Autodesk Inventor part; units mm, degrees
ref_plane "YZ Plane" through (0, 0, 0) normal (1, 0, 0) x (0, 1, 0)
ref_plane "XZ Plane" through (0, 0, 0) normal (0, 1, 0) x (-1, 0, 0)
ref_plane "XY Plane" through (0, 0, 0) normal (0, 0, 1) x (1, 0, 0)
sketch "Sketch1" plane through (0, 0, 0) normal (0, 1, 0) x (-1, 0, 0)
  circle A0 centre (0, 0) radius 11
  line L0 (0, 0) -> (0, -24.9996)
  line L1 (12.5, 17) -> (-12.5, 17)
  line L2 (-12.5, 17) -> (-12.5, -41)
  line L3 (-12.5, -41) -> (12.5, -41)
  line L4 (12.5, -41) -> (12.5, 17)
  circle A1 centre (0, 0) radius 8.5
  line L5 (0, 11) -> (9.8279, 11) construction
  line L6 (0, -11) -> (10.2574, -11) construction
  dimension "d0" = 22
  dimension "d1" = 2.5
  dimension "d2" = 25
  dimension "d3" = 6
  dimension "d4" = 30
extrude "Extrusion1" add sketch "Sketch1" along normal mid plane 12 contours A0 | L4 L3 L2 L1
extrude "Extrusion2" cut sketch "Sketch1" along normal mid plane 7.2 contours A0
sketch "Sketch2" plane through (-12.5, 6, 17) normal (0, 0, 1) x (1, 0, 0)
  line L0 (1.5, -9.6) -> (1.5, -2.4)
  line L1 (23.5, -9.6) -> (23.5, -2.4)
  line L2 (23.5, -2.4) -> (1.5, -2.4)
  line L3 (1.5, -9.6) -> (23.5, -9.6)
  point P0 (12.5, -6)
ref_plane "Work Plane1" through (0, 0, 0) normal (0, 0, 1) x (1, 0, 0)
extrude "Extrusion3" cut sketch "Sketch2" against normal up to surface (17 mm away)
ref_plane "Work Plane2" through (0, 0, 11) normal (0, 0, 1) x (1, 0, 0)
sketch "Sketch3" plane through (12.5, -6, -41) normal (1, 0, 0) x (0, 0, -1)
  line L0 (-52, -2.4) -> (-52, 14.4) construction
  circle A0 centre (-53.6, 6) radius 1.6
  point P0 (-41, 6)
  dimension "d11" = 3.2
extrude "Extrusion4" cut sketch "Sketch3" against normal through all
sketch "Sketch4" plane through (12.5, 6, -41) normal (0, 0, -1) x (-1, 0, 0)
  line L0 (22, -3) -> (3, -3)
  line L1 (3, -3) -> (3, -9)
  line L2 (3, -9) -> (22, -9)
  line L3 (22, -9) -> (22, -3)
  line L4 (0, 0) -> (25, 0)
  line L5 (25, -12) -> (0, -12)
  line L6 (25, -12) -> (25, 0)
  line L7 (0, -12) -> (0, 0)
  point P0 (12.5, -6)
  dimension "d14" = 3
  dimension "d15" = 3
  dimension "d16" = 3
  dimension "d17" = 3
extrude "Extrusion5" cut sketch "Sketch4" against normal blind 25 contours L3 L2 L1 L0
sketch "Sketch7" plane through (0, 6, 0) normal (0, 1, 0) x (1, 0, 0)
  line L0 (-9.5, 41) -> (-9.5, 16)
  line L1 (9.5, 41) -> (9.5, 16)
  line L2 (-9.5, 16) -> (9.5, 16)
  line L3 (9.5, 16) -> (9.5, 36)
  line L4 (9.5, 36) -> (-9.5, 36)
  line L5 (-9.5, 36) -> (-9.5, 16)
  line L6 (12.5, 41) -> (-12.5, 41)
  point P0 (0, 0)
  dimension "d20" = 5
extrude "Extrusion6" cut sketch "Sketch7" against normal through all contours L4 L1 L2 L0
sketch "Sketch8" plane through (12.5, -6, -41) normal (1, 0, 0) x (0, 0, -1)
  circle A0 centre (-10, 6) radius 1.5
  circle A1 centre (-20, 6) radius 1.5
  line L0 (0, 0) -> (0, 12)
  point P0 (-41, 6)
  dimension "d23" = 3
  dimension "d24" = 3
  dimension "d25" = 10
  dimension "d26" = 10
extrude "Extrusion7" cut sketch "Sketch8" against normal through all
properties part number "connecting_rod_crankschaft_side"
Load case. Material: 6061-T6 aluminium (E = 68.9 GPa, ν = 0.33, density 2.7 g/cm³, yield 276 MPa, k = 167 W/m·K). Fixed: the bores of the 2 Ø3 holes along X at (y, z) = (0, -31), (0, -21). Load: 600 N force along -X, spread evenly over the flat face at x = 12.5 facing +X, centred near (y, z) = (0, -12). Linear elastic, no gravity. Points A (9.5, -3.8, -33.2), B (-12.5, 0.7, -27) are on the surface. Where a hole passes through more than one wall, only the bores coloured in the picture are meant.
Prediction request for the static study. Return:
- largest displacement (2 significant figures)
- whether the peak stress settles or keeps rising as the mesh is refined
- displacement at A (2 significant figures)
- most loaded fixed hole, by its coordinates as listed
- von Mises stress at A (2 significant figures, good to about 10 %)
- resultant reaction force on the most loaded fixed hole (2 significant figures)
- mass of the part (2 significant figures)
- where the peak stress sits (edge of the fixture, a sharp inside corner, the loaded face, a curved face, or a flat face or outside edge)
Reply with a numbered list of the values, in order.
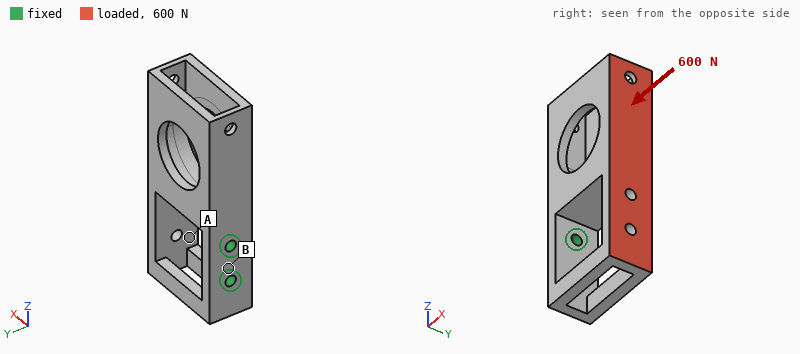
1. 0.29 mm
2. keeps rising
3. 0.13 mm
4. (0, -21)
5. 63 MPa
6. 710 N
7. 19 g
8. edge of the fixture
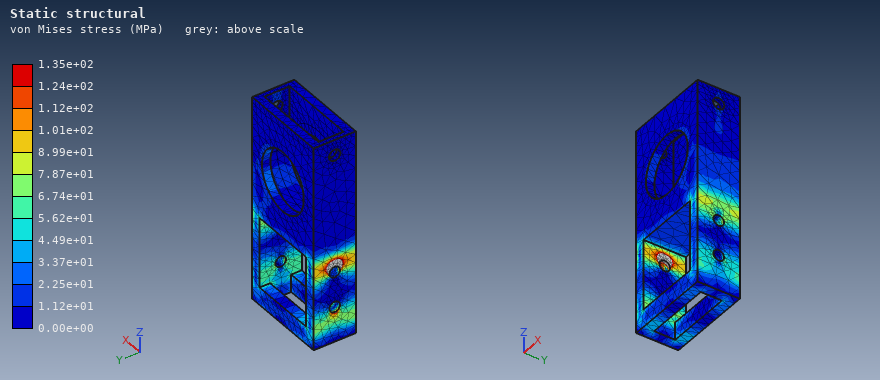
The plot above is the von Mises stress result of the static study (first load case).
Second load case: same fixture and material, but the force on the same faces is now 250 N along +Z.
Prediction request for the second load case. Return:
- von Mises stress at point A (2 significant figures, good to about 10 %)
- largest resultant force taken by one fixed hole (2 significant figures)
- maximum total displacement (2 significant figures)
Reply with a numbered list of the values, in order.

1. 55 MPa
2. 270 N
3. 0.26 mm
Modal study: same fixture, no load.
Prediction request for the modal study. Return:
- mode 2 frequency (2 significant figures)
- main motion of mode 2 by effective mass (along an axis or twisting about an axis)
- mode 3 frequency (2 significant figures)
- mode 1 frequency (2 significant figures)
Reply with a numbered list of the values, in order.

1. 2100 Hz
2. along Y
3. 3500 Hz
4. 1700 Hz
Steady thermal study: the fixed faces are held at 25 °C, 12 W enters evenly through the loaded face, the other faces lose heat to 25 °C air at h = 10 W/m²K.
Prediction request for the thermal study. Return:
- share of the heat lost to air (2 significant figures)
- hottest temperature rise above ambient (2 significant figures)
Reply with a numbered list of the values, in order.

1. 6.1 %
2. 23 K
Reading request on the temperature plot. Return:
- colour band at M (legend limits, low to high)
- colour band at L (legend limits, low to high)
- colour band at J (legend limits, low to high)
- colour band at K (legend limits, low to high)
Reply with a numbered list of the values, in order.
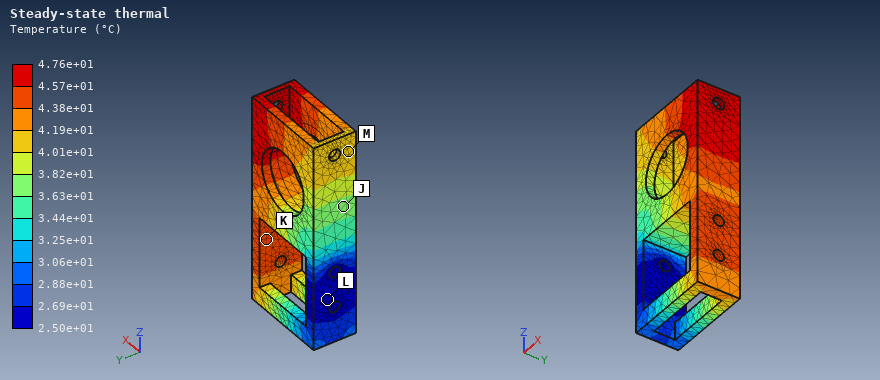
1. 4.01e+01 to 4.19e+01 °C
2. 2.50e+01 to 2.69e+01 °C
3. 3.63e+01 to 3.82e+01 °C
4. 4.38e+01 to 4.57e+01 °C
